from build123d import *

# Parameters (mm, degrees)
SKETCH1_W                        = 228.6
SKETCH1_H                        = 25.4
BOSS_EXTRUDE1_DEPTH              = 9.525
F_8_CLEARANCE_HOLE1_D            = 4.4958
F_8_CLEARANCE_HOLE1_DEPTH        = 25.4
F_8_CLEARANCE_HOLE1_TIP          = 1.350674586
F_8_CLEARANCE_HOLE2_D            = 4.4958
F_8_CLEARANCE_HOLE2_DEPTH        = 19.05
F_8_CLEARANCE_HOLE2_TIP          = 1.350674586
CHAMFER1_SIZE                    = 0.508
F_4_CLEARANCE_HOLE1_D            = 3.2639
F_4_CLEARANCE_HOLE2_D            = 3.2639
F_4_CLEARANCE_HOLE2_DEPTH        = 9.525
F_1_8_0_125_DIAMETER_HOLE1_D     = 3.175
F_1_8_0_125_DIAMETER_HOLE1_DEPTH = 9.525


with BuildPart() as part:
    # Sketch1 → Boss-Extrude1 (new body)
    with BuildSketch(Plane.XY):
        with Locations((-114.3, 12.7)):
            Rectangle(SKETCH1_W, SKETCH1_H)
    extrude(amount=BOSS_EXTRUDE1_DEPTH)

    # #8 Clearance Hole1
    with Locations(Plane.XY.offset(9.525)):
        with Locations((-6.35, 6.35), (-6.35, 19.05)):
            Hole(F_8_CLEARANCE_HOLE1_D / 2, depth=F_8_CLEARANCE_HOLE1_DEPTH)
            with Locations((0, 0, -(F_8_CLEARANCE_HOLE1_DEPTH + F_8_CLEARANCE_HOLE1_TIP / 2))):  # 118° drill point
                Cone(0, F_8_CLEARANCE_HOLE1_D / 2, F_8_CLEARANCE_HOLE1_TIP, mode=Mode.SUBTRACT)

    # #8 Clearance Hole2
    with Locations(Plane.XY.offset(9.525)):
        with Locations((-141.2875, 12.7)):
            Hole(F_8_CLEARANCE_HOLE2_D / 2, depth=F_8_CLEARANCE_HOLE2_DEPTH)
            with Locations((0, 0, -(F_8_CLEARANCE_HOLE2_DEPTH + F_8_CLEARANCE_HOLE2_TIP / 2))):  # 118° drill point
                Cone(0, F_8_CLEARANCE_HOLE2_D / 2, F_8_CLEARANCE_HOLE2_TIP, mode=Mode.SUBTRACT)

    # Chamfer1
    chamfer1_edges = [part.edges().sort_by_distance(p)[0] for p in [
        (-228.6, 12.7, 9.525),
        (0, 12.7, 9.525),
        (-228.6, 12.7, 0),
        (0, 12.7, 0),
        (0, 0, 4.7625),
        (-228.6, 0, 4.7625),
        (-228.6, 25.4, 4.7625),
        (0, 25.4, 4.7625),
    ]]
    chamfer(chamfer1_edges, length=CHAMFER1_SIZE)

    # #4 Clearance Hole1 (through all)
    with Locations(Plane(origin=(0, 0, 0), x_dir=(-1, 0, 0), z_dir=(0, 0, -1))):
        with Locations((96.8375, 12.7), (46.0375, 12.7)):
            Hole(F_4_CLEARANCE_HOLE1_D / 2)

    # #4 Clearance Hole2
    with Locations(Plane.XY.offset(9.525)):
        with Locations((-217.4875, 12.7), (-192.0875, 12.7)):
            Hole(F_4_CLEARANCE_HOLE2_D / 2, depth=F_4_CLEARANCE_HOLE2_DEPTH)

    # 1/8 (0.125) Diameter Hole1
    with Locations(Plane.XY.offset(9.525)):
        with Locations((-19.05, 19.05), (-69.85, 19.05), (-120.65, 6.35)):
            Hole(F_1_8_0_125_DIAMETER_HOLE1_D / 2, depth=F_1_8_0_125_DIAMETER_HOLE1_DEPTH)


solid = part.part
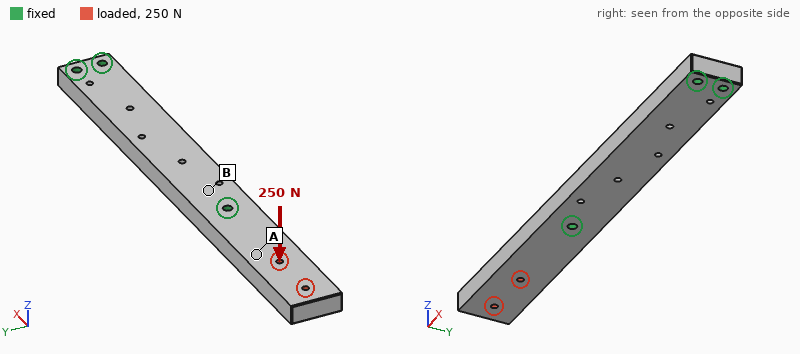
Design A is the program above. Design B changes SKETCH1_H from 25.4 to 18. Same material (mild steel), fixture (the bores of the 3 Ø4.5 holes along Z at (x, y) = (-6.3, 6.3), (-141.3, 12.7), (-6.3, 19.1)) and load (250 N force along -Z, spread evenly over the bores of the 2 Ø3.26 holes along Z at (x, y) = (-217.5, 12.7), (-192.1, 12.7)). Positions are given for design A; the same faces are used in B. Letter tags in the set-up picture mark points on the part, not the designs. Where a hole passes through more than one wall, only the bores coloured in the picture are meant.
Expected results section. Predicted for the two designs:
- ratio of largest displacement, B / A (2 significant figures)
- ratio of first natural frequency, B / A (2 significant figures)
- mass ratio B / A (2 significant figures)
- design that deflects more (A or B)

1.3
1.0
0.70
B
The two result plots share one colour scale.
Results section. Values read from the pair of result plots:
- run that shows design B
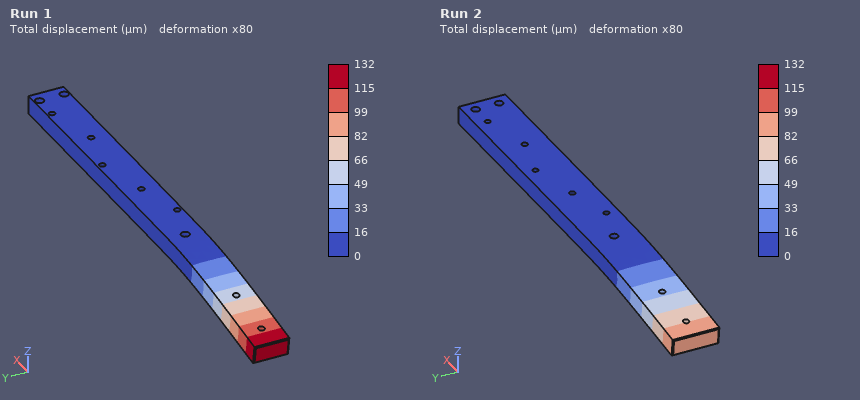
Run 1
